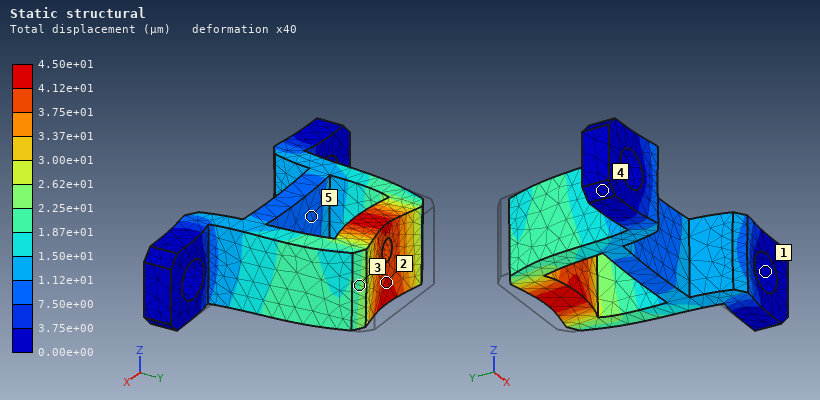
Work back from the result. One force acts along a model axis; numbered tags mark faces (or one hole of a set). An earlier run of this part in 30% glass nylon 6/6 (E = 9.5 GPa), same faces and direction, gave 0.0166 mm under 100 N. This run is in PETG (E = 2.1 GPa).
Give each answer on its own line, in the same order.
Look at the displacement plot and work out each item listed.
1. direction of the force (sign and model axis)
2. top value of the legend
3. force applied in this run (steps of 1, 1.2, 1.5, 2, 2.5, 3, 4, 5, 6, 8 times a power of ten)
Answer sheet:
-Y
4.50e+01 µm
60 N
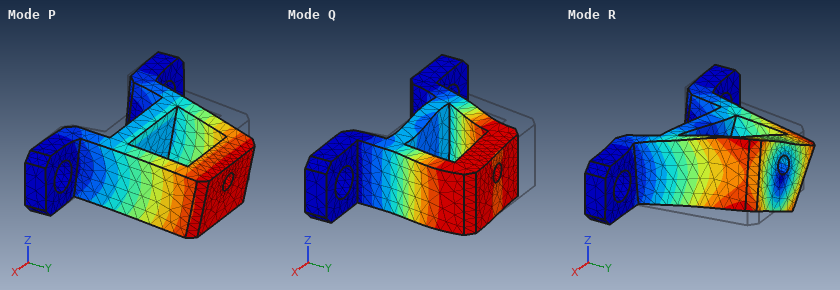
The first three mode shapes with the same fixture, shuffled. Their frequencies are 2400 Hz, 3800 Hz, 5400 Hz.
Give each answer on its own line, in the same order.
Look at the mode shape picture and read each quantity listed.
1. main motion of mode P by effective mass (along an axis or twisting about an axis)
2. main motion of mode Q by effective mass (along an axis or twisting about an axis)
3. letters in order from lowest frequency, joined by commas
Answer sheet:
along Z
along X
P, Q, R
